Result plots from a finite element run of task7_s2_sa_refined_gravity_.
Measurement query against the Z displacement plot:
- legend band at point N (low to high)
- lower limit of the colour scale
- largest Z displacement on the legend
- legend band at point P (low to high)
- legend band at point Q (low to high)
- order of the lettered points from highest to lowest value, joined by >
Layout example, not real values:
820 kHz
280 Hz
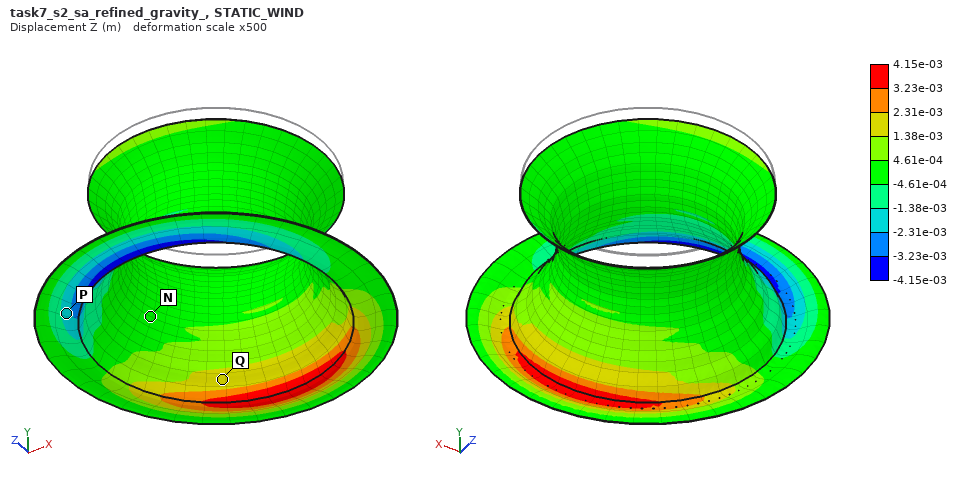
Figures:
-4.61e-04 to 4.61e-04 m
-4.15e-03 m
4.15e-03 m
-2.31e-03 to -1.38e-03 m
1.38e-03 to 2.31e-03 m
Q > N > P
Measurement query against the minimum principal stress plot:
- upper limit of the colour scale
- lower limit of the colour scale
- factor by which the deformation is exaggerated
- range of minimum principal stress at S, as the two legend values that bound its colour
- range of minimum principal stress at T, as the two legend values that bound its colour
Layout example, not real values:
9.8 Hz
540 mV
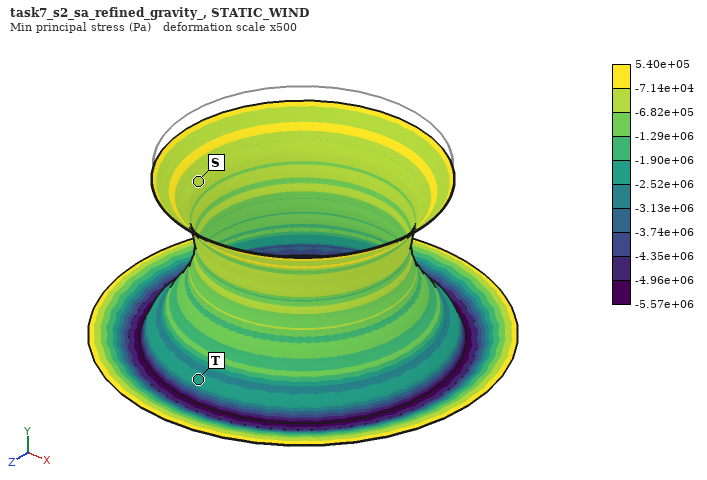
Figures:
5.40e+05 Pa
-5.57e+06 Pa
500
-6.82e+05 to -7.14e+04 Pa
-2.52e+06 to -1.90e+06 Pa
